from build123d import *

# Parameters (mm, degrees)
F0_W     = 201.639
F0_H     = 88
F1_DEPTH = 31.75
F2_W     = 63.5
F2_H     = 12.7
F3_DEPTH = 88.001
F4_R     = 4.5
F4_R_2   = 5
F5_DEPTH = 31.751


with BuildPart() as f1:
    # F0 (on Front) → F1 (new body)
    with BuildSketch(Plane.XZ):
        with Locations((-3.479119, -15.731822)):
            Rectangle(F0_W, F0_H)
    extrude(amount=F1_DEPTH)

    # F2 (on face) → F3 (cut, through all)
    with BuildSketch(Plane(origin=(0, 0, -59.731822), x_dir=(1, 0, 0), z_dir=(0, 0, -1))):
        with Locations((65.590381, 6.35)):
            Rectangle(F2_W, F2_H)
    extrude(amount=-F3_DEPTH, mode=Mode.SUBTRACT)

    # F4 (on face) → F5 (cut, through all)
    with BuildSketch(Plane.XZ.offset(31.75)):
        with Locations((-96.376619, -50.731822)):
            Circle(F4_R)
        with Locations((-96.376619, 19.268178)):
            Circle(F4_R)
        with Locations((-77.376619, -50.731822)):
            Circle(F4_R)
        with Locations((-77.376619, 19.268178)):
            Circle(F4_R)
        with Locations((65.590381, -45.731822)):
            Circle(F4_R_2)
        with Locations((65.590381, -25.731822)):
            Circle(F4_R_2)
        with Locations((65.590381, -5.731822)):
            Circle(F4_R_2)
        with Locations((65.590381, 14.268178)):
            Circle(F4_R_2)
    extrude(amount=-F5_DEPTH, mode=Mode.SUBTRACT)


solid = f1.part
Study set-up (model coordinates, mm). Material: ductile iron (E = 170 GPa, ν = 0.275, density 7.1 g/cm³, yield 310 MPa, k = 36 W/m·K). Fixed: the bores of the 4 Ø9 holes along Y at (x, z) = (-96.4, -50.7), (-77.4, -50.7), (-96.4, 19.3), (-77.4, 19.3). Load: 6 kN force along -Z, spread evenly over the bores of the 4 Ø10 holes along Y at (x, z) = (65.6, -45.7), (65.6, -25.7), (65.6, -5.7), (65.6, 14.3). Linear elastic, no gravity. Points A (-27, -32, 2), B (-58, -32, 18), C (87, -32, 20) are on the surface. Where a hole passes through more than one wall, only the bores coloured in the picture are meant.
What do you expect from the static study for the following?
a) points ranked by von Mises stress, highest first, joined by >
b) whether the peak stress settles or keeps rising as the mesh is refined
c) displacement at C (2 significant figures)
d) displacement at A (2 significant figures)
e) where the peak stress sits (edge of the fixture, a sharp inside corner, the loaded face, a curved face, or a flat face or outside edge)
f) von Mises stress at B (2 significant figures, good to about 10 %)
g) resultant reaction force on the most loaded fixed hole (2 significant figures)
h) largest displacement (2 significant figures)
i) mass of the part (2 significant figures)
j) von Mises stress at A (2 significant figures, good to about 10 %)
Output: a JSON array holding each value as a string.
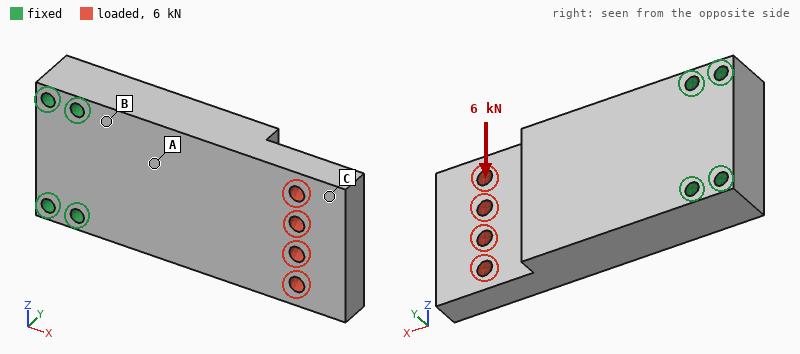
["B > A > C", "keeps rising", "32 µm", "5.5 µm", "edge of the fixture", "14 MPa", "11 kN", "35 µm", "3.4 kg", "8.8 MPa"]
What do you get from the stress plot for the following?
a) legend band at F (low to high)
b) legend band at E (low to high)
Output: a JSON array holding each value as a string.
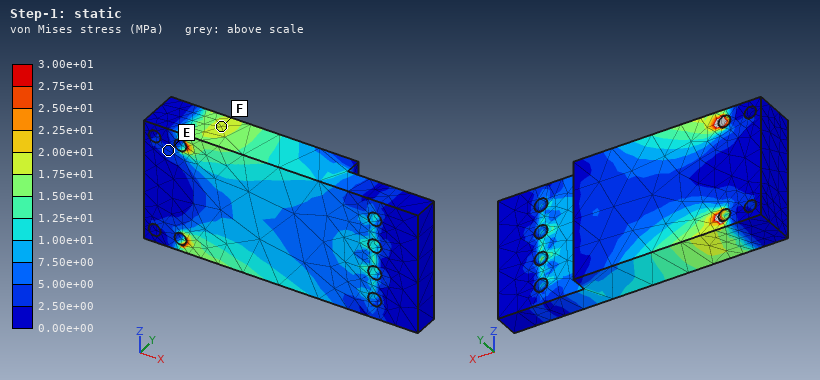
["1.75e+01 to 2.00e+01 MPa", "2.50e+00 to 5.00e+00 MPa"]
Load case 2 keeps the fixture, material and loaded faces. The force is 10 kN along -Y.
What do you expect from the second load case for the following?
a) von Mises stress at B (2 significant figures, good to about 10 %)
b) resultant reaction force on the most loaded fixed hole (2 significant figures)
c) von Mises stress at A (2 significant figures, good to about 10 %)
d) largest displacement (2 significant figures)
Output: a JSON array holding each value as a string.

["99 MPa", "11 kN", "62 MPa", "0.41 mm"]
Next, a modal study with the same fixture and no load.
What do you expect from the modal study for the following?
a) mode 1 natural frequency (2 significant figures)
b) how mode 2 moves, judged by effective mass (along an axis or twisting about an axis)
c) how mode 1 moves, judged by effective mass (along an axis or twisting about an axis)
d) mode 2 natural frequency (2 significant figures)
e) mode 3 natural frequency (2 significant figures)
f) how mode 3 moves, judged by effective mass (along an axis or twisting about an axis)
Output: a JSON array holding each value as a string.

["920 Hz", "along Z", "along Y", "2400 Hz", "3100 Hz", "twisting about X"]
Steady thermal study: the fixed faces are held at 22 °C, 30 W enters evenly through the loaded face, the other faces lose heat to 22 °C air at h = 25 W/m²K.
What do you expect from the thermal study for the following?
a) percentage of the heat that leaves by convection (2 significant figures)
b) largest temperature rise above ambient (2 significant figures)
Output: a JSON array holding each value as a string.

["55 %", "33 K"]
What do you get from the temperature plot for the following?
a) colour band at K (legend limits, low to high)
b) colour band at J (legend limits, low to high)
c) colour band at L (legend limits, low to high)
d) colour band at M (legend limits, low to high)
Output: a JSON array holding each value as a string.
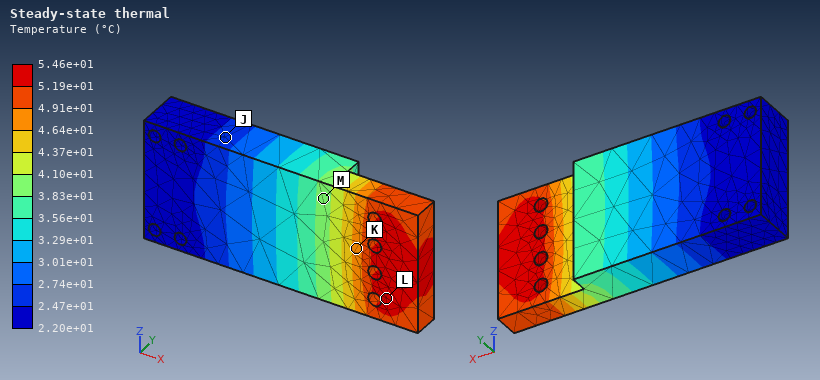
["4.64e+01 to 4.91e+01 °C", "2.47e+01 to 2.74e+01 °C", "5.19e+01 to 5.46e+01 °C", "3.83e+01 to 4.10e+01 °C"]
